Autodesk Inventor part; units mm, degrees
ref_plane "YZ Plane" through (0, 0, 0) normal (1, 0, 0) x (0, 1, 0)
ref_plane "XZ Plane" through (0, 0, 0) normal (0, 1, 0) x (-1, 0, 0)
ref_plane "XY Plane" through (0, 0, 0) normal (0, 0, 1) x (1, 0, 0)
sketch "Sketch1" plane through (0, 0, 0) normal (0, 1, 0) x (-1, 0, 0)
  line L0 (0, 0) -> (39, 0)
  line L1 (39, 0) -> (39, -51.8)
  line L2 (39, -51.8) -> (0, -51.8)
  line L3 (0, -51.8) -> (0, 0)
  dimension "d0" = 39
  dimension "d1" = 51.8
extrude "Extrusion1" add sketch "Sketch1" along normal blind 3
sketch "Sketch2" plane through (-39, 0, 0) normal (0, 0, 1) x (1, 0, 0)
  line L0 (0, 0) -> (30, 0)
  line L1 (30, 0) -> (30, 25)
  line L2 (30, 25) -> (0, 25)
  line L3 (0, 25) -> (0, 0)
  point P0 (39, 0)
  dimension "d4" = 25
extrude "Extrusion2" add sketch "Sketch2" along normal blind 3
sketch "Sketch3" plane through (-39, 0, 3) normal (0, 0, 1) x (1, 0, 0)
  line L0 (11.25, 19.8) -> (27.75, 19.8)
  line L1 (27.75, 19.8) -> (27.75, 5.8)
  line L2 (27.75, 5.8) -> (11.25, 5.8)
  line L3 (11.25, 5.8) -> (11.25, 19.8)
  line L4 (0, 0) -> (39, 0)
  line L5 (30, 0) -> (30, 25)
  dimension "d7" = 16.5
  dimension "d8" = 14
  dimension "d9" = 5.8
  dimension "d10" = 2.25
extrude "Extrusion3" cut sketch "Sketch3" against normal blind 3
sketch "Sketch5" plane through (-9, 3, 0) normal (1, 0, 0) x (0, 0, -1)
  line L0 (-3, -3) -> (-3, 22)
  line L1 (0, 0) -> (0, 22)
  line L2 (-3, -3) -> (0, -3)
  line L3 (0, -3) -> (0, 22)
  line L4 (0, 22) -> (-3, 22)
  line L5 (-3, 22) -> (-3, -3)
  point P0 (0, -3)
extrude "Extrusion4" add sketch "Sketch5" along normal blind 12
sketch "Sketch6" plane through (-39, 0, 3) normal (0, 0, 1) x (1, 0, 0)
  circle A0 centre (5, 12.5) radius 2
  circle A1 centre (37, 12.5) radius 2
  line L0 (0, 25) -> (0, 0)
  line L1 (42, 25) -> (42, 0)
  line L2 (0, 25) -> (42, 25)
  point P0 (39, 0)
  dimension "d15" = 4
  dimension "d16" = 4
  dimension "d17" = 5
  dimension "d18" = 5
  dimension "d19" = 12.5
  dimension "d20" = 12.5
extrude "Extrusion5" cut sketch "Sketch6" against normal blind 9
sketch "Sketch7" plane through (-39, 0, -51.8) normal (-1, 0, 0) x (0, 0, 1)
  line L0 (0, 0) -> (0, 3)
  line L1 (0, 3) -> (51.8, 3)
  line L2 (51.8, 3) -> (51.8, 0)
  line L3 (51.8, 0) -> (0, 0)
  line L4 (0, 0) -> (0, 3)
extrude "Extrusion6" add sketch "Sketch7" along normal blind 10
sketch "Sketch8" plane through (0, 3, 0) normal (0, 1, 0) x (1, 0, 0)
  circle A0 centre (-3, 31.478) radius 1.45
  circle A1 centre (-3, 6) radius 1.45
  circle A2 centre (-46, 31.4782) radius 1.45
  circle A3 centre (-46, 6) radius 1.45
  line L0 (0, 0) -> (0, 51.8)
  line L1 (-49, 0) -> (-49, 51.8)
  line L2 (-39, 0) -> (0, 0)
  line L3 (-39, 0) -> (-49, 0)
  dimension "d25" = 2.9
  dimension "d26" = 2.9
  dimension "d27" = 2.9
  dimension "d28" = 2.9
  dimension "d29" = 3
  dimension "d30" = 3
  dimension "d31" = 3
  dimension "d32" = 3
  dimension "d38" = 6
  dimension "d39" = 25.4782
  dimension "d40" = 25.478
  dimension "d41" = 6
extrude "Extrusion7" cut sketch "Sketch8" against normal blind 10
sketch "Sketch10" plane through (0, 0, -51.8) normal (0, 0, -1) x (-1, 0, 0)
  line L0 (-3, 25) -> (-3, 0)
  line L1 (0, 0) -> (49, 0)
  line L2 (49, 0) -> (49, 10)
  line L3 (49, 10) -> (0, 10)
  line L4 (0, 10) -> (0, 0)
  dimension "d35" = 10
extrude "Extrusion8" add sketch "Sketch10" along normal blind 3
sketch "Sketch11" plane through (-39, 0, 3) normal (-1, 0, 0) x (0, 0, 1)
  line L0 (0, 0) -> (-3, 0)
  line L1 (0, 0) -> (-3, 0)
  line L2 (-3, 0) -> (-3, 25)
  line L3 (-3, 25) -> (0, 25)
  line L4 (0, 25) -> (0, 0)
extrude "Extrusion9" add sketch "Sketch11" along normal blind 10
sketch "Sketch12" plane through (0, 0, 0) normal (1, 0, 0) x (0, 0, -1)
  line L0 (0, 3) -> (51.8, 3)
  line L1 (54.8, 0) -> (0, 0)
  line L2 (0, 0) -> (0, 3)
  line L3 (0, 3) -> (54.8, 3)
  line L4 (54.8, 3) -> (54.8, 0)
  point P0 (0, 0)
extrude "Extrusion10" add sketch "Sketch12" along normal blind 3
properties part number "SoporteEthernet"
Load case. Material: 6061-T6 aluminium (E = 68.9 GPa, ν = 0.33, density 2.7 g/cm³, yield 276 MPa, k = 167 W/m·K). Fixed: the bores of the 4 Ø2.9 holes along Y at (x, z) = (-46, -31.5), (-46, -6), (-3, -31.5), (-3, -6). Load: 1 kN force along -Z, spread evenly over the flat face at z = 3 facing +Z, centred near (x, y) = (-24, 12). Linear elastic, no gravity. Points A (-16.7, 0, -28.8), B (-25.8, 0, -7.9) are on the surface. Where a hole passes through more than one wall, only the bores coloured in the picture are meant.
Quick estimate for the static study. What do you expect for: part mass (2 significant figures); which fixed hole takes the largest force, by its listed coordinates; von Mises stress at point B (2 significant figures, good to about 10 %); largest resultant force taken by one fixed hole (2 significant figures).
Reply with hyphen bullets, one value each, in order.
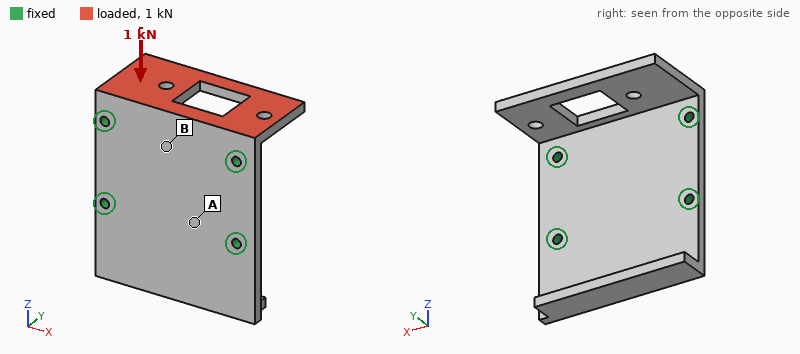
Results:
- 34 g
- (-3, -6)
- 56 MPa
- 370 N
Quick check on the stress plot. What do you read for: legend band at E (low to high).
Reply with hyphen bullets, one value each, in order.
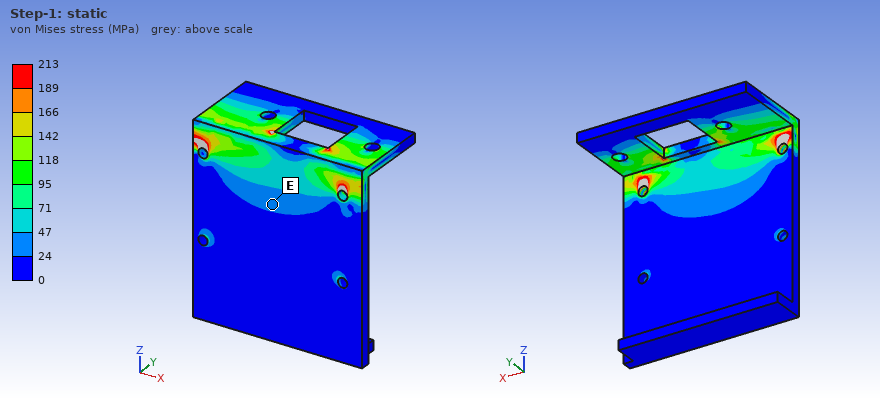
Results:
- 24 to 47 MPa
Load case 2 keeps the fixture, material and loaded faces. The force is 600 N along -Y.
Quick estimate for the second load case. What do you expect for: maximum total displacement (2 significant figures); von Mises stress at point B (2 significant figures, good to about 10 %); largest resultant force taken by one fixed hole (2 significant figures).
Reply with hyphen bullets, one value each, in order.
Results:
- 0.13 mm
- 17 MPa
- 340 N
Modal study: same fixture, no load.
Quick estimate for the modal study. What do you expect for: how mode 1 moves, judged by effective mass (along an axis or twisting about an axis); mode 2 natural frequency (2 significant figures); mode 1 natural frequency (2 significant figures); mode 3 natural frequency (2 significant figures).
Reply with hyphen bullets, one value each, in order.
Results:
- along Y
- 2800 Hz
- 2700 Hz
- 4500 Hz
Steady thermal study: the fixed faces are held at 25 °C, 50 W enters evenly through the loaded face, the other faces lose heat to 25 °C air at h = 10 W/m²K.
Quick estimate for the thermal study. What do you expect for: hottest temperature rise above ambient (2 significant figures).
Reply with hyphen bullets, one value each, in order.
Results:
- 58 K
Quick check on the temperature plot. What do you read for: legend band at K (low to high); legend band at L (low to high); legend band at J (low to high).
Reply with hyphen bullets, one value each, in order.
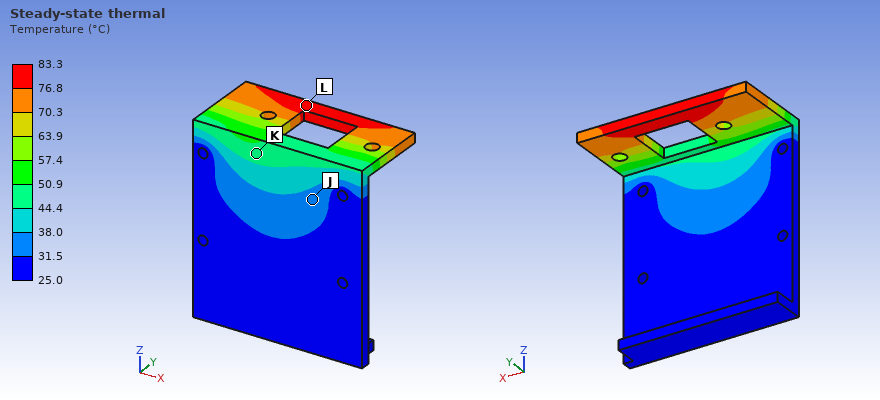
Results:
- 44.4 to 50.9 °C
- 76.8 to 83.3 °C
- 31.5 to 38.0 °C
